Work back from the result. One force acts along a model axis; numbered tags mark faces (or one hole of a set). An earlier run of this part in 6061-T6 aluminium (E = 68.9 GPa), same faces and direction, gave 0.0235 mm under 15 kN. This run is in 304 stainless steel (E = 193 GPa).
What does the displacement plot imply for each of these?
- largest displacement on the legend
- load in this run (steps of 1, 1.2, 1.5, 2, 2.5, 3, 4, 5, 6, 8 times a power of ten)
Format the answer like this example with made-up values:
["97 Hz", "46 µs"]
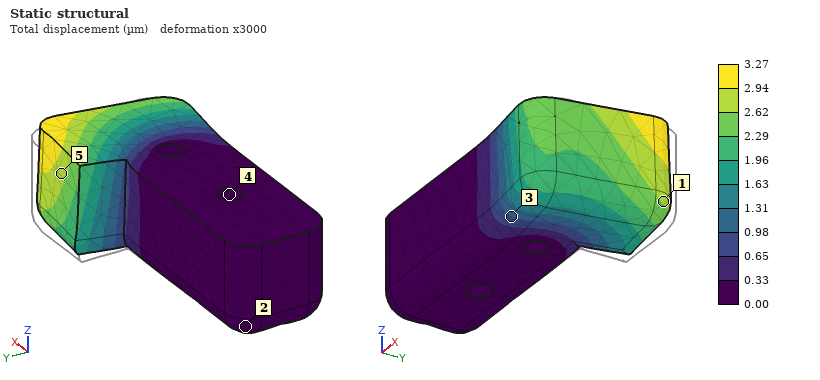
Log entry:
["3.27 µm", "6 kN"]
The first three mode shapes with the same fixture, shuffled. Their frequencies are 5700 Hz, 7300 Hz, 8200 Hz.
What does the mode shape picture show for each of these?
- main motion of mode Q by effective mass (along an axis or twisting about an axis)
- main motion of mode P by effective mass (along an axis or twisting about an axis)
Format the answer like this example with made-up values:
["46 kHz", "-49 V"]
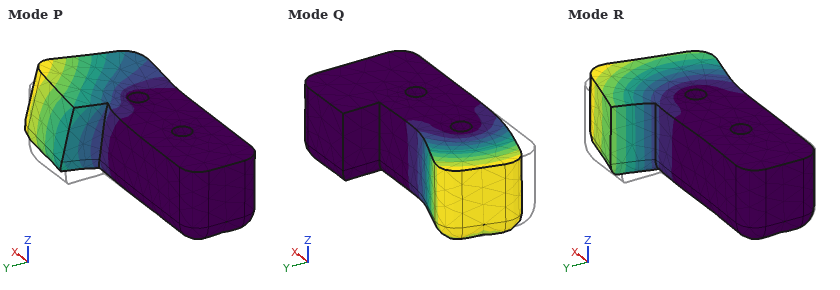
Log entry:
["along Y", "along Z"]
